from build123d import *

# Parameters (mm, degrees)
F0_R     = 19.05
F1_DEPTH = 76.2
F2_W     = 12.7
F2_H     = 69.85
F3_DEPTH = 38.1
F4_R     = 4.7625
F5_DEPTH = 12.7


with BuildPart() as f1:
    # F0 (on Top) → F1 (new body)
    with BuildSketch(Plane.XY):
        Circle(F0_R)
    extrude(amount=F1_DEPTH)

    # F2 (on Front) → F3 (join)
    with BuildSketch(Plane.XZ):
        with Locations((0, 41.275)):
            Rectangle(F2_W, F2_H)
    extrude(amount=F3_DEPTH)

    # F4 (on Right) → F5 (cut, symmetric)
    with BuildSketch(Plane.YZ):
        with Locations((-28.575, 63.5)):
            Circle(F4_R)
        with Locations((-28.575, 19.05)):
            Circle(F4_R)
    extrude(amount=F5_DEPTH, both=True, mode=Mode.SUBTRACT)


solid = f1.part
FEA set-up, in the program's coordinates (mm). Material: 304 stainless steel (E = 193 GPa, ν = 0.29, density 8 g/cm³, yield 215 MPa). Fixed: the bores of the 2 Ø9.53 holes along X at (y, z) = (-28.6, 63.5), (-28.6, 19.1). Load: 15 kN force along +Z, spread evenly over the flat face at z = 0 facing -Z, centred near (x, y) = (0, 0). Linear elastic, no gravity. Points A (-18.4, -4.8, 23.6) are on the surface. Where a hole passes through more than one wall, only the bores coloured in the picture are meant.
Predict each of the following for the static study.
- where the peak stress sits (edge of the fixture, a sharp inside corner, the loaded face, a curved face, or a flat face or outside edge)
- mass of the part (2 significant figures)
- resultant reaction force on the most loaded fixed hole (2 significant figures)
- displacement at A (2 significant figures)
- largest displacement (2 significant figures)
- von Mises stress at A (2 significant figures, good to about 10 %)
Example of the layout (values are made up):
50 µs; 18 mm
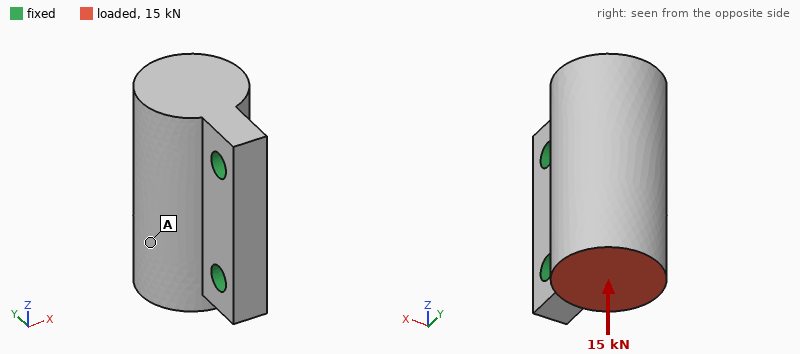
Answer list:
edge of the fixture; 820 g; 11 kN; 6.6 µm; 13 µm; 11 MPa
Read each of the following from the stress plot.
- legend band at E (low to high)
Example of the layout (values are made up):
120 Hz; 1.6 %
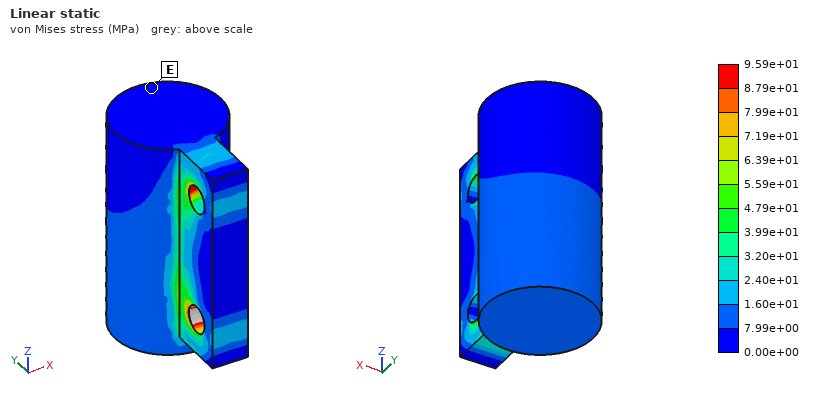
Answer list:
0.00e+00 to 7.99e+00 MPa
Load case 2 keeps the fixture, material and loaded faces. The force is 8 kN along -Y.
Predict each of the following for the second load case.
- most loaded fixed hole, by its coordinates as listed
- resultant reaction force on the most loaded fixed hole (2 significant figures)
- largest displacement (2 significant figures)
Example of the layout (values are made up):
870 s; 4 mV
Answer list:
(-28.6, 19.1); 11 kN; 11 µm
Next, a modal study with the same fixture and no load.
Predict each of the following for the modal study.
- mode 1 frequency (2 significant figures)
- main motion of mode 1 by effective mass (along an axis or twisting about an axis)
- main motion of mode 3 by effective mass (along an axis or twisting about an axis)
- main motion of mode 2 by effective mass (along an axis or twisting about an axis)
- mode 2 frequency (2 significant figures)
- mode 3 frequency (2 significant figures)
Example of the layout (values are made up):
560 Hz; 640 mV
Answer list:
2900 Hz; along X; along Z; twisting about Y; 7600 Hz; 8500 Hz
